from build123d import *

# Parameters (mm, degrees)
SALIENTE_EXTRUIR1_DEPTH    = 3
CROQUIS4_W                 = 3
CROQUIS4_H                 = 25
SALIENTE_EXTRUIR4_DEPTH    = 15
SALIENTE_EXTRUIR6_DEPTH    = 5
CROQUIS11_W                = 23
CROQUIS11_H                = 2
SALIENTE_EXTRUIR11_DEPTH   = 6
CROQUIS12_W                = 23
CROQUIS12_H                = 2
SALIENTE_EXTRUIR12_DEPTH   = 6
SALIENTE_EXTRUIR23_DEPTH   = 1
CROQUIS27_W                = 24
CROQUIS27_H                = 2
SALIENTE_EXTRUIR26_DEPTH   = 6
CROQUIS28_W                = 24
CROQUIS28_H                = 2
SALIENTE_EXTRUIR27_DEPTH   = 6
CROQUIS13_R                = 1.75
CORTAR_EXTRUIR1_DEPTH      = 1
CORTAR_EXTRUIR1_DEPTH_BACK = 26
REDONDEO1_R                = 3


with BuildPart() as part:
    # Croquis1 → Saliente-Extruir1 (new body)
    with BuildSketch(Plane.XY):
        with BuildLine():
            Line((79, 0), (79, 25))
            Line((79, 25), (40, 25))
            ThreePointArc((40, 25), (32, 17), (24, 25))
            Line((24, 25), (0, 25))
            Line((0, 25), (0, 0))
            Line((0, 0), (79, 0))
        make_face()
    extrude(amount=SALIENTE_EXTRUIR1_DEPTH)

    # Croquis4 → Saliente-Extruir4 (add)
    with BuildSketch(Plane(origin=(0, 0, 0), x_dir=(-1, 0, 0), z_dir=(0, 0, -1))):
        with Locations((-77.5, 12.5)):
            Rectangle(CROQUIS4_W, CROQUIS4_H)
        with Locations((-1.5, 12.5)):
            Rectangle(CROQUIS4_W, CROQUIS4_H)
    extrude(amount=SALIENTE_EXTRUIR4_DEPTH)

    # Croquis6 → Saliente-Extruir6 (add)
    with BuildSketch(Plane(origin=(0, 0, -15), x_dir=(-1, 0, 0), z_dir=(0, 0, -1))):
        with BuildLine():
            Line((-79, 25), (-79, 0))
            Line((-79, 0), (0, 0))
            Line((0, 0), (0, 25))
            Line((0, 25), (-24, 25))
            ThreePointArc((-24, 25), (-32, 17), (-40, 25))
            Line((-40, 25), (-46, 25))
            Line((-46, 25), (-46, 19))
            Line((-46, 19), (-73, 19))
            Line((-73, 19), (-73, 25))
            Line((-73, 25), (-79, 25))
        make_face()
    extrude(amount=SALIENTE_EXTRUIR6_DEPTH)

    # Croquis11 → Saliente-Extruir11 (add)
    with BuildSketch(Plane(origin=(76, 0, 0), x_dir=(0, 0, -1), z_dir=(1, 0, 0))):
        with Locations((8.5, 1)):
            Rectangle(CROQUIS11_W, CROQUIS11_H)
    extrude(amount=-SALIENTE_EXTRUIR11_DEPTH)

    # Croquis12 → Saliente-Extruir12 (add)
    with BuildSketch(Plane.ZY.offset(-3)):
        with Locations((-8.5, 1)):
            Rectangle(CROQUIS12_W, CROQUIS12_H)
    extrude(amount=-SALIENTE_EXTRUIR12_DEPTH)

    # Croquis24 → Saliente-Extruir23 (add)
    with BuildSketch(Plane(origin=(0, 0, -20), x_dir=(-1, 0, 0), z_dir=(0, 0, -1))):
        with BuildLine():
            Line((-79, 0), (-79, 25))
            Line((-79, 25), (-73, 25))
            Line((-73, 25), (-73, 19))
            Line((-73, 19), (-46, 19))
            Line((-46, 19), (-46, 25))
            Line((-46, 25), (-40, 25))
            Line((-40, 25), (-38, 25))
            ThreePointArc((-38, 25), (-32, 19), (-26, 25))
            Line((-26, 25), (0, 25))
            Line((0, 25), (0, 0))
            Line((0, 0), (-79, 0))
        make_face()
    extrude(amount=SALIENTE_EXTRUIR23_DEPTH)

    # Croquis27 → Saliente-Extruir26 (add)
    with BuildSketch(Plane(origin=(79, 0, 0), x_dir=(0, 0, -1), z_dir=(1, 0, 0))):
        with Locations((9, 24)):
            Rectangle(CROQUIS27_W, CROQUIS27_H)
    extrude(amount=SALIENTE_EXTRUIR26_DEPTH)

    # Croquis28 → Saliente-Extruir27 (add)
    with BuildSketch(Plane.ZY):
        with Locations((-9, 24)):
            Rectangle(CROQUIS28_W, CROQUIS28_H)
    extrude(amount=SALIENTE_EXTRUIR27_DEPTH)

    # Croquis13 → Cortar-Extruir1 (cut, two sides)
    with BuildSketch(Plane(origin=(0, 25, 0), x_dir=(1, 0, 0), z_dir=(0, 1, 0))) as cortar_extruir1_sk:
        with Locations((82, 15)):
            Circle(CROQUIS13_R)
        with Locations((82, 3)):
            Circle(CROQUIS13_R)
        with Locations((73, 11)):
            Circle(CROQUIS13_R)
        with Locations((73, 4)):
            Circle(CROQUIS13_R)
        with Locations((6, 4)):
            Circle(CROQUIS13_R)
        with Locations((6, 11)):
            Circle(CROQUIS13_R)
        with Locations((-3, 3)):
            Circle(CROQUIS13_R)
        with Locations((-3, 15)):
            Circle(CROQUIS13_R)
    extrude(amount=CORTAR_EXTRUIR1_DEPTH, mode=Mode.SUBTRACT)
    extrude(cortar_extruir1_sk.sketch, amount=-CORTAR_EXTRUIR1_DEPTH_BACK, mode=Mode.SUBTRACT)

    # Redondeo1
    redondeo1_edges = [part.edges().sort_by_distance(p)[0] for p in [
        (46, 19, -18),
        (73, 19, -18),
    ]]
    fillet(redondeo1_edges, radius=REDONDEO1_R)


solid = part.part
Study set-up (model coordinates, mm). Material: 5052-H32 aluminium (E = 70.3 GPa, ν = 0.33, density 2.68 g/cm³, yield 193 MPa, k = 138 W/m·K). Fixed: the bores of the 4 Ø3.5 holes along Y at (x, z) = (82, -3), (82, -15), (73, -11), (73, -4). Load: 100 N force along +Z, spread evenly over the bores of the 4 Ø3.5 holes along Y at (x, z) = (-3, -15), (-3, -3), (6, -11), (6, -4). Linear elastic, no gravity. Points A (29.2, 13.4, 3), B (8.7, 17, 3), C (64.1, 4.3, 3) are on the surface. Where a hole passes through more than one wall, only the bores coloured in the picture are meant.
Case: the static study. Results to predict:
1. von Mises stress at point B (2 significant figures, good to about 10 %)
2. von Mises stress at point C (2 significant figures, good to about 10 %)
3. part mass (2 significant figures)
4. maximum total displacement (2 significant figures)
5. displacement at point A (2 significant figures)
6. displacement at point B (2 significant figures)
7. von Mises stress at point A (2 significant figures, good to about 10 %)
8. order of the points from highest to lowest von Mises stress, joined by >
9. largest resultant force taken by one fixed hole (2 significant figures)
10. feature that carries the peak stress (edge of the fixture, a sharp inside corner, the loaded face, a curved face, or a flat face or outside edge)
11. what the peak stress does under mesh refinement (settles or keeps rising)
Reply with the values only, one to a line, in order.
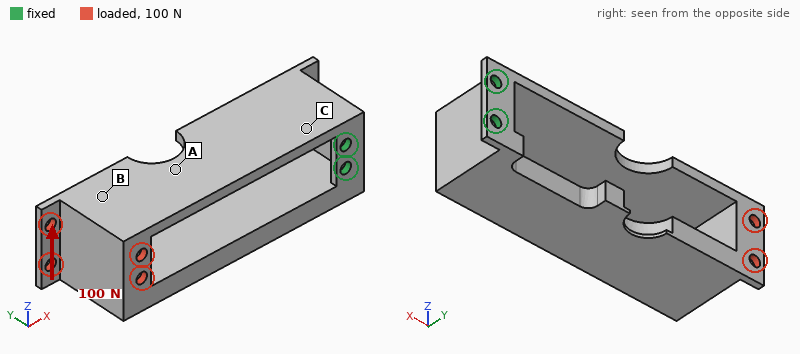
12 MPa
19 MPa
51 g
0.24 mm
0.16 mm
0.22 mm
5.9 MPa
C > B > A
340 N
edge of the fixture
keeps rising
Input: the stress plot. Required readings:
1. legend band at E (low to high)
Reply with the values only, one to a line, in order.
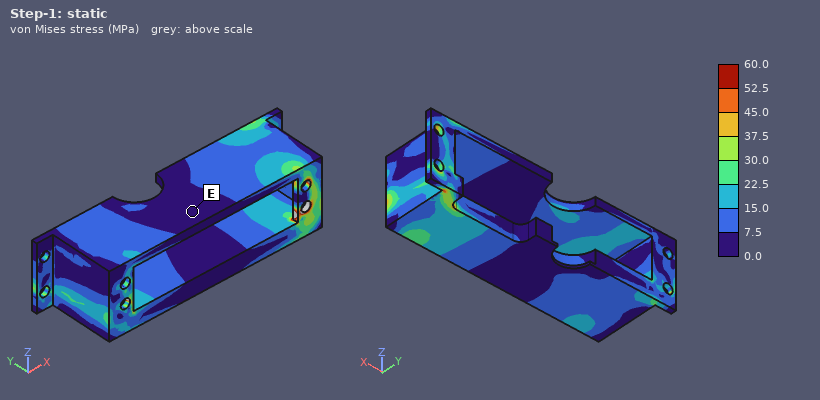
0.0 to 7.5 MPa
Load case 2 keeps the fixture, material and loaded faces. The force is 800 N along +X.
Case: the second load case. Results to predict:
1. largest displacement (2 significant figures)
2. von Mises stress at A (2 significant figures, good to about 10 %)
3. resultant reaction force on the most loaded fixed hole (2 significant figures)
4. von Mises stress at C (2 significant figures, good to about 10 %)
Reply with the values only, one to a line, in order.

31 µm
7.1 MPa
230 N
5.4 MPa
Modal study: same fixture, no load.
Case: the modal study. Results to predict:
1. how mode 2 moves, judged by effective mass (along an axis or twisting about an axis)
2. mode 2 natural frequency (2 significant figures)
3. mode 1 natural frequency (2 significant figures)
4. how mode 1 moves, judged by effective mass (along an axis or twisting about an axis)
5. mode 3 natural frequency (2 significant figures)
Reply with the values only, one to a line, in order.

along Y
1800 Hz
750 Hz
along Z
2900 Hz
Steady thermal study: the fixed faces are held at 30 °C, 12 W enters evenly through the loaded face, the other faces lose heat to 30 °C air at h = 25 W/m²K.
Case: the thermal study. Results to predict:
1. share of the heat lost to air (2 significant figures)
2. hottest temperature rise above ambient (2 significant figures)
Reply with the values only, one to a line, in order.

36 %
36 K
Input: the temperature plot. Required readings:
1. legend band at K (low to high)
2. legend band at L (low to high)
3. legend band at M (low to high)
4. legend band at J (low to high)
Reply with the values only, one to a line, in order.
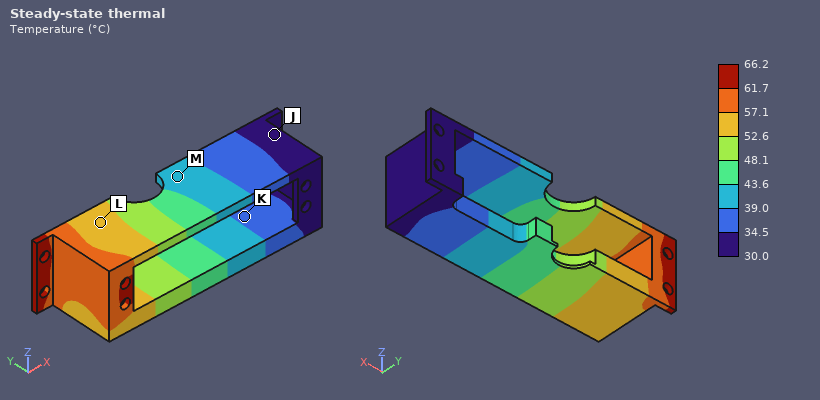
34.5 to 39.0 °C
52.6 to 57.1 °C
39.0 to 43.6 °C
30.0 to 34.5 °C
